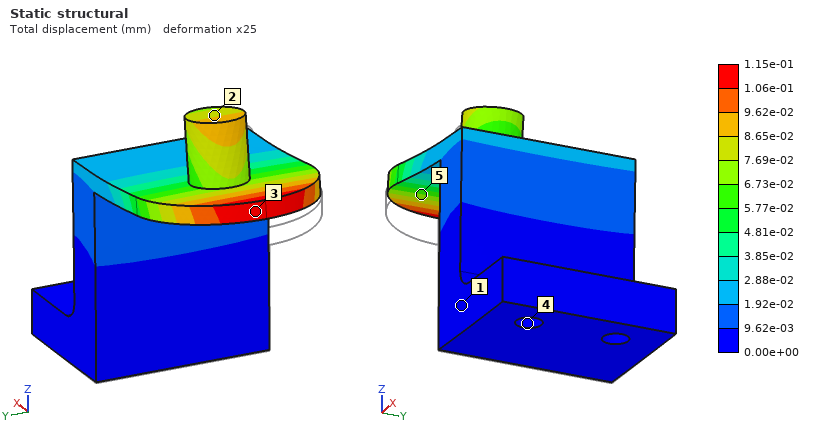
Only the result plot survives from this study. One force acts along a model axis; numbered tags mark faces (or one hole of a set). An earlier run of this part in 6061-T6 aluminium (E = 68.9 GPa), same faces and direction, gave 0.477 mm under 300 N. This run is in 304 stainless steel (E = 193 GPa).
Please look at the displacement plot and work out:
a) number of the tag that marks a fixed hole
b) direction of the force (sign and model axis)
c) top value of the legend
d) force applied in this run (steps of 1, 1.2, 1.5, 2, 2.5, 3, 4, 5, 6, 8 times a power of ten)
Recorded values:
4
+Z
1.15e-01 mm
200 N
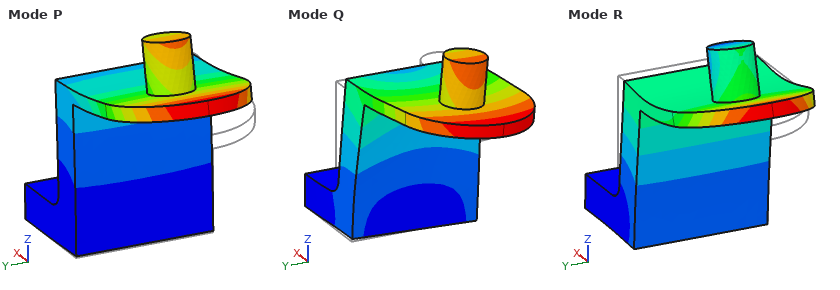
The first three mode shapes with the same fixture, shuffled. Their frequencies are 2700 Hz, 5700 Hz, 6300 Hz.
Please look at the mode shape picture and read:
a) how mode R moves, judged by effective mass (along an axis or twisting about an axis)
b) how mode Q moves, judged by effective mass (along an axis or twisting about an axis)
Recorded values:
along X
along Y
